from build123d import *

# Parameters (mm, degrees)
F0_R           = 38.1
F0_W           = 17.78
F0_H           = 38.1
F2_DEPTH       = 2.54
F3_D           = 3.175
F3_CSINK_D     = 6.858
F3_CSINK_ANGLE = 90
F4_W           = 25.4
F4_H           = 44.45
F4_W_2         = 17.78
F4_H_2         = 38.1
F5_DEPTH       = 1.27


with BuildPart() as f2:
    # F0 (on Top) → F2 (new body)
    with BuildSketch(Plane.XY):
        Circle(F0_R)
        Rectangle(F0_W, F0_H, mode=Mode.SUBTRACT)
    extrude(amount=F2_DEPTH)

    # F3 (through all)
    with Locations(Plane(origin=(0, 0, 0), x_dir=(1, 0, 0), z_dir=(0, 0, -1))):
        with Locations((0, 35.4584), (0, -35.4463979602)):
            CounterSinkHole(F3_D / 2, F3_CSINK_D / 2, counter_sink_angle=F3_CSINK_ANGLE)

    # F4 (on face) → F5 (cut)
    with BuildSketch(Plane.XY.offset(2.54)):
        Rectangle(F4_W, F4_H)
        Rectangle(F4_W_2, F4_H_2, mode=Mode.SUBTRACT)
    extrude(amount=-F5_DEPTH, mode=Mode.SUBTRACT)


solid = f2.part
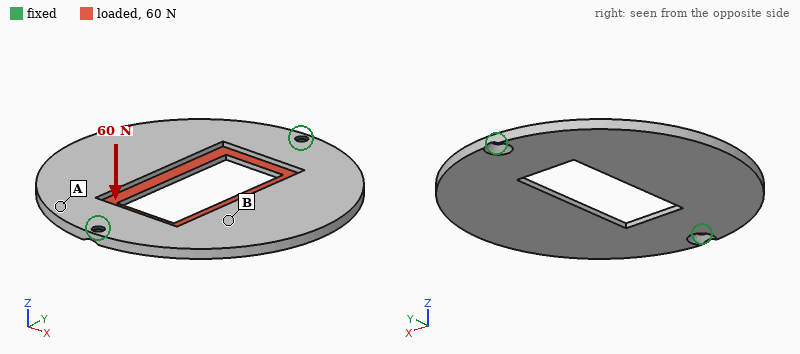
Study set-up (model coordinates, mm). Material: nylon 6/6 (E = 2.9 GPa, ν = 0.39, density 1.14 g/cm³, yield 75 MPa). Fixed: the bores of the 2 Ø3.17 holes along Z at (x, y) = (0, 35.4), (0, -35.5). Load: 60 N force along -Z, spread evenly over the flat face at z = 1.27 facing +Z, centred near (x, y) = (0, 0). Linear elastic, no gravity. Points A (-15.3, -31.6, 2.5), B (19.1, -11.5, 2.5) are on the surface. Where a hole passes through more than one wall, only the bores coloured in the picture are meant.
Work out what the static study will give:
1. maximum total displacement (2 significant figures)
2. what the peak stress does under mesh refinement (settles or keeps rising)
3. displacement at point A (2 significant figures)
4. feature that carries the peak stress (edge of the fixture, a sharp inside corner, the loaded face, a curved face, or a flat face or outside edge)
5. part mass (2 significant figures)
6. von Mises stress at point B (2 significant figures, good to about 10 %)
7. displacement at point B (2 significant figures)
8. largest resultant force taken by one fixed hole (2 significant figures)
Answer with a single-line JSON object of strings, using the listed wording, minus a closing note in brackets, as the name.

{"maximum total displacement": "1.2 mm", "what the peak stress does under mesh refinement": "keeps rising", "displacement at point A": "0.21 mm", "feature that carries the peak stress": "edge of the fixture", "part mass": "10 g", "von Mises stress at point B": "6.5 MPa", "displacement at point B": "0.88 mm", "largest resultant force taken by one fixed hole": "73 N"}
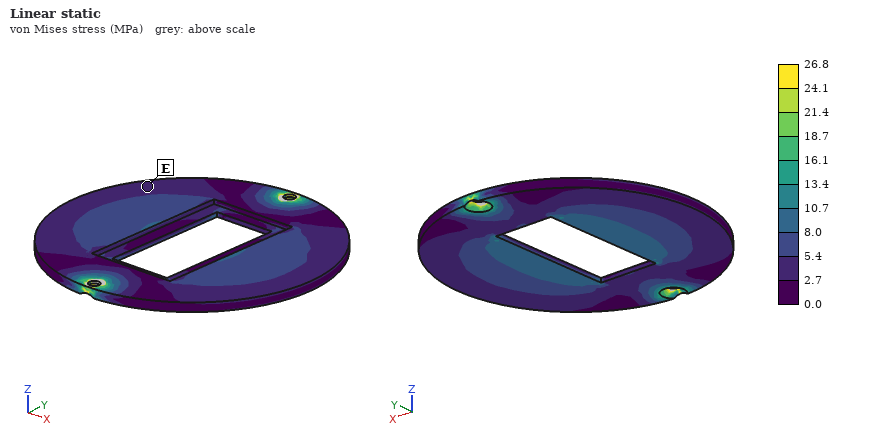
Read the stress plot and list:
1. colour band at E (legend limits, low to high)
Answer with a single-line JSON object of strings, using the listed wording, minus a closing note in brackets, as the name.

{"colour band at E": "2.7 to 5.4 MPa"}
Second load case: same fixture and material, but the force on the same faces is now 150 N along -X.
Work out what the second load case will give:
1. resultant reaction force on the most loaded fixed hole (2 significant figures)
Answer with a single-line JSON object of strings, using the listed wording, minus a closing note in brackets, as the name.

{"resultant reaction force on the most loaded fixed hole": "75 N"}
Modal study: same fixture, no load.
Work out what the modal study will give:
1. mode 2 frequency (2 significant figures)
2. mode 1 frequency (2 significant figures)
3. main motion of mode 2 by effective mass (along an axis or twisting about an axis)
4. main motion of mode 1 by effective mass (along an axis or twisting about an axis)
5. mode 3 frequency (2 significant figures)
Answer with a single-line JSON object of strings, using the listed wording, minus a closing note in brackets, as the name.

{"mode 2 frequency": "330 Hz", "mode 1 frequency": "200 Hz", "main motion of mode 2 by effective mass": "along Z", "main motion of mode 1 by effective mass": "twisting about Y", "mode 3 frequency": "750 Hz"}
